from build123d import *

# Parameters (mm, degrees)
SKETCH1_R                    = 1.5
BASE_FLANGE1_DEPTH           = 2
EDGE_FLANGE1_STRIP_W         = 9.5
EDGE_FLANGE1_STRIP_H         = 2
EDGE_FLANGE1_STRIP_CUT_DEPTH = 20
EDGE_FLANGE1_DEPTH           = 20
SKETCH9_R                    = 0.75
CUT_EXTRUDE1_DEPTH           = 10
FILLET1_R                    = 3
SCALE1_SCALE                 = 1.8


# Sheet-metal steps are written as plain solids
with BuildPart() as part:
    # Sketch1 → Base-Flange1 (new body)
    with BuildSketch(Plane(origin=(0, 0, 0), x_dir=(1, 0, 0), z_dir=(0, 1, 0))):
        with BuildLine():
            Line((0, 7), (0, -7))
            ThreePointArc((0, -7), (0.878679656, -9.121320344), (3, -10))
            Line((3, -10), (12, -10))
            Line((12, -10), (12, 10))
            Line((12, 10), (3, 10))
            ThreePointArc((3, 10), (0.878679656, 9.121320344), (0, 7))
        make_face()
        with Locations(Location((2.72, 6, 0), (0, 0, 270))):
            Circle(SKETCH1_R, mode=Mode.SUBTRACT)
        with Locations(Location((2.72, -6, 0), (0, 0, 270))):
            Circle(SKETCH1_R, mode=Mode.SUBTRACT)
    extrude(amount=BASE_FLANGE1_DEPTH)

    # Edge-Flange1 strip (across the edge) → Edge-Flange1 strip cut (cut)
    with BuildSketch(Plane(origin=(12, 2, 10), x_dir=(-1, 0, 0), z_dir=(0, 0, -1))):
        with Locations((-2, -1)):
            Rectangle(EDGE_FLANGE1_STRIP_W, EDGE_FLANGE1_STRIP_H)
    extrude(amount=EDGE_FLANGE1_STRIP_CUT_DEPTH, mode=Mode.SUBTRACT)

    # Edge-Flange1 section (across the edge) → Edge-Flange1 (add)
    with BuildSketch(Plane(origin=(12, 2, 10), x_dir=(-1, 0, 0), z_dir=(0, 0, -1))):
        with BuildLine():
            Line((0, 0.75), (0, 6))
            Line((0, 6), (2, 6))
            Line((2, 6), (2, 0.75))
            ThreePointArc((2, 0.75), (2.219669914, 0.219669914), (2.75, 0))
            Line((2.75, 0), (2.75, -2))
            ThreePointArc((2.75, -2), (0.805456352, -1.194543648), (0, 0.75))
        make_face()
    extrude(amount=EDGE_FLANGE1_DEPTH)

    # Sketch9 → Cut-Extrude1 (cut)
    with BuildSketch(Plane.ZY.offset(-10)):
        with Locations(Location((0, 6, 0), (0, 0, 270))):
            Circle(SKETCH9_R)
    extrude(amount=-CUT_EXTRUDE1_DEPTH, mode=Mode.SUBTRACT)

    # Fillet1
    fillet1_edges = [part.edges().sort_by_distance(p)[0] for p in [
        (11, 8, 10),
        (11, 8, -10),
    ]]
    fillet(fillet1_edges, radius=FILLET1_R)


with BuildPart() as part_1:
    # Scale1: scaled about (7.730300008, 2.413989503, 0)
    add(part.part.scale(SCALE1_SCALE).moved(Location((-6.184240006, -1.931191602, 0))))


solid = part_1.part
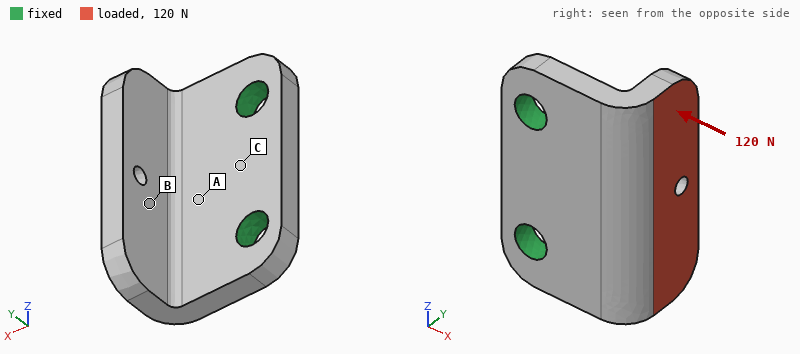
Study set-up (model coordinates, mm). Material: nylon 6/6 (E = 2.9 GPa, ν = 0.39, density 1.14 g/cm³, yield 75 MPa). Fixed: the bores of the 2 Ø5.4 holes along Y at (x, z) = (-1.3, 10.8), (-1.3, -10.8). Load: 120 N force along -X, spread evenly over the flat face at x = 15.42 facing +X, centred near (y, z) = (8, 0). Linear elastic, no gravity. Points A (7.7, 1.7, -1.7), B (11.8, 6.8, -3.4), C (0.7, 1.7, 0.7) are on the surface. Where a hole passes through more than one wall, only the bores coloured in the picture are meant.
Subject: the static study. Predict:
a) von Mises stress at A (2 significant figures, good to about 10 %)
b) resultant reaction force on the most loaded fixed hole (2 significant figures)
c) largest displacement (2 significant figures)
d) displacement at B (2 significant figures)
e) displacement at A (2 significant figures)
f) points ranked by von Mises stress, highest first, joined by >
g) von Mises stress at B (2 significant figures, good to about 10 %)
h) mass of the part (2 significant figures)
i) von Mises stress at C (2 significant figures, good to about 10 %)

11 MPa
62 N
0.49 mm
0.26 mm
0.079 mm
A > C > B
2.7 MPa
4.3 g
5.8 MPa
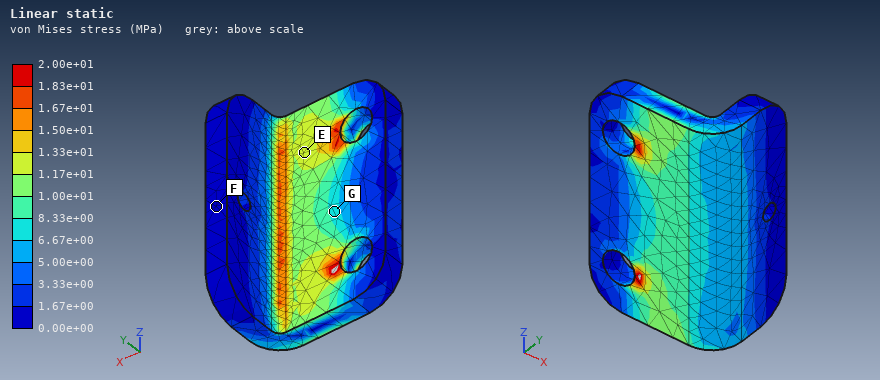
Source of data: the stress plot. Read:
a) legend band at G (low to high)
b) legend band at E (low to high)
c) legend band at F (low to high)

6.67e+00 to 8.33e+00 MPa
1.17e+01 to 1.33e+01 MPa
0.00e+00 to 1.67e+00 MPa
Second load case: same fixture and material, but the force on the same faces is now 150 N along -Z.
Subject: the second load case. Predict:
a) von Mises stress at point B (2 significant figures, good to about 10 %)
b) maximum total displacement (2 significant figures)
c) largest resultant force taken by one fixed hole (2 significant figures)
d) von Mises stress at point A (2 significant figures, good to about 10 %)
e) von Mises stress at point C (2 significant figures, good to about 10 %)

3.2 MPa
0.17 mm
130 N
7.1 MPa
2.9 MPa
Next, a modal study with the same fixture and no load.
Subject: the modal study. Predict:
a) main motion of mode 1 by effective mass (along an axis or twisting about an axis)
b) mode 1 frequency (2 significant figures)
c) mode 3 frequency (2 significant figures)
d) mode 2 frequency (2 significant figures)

along Y
1900 Hz
5500 Hz
3000 Hz
